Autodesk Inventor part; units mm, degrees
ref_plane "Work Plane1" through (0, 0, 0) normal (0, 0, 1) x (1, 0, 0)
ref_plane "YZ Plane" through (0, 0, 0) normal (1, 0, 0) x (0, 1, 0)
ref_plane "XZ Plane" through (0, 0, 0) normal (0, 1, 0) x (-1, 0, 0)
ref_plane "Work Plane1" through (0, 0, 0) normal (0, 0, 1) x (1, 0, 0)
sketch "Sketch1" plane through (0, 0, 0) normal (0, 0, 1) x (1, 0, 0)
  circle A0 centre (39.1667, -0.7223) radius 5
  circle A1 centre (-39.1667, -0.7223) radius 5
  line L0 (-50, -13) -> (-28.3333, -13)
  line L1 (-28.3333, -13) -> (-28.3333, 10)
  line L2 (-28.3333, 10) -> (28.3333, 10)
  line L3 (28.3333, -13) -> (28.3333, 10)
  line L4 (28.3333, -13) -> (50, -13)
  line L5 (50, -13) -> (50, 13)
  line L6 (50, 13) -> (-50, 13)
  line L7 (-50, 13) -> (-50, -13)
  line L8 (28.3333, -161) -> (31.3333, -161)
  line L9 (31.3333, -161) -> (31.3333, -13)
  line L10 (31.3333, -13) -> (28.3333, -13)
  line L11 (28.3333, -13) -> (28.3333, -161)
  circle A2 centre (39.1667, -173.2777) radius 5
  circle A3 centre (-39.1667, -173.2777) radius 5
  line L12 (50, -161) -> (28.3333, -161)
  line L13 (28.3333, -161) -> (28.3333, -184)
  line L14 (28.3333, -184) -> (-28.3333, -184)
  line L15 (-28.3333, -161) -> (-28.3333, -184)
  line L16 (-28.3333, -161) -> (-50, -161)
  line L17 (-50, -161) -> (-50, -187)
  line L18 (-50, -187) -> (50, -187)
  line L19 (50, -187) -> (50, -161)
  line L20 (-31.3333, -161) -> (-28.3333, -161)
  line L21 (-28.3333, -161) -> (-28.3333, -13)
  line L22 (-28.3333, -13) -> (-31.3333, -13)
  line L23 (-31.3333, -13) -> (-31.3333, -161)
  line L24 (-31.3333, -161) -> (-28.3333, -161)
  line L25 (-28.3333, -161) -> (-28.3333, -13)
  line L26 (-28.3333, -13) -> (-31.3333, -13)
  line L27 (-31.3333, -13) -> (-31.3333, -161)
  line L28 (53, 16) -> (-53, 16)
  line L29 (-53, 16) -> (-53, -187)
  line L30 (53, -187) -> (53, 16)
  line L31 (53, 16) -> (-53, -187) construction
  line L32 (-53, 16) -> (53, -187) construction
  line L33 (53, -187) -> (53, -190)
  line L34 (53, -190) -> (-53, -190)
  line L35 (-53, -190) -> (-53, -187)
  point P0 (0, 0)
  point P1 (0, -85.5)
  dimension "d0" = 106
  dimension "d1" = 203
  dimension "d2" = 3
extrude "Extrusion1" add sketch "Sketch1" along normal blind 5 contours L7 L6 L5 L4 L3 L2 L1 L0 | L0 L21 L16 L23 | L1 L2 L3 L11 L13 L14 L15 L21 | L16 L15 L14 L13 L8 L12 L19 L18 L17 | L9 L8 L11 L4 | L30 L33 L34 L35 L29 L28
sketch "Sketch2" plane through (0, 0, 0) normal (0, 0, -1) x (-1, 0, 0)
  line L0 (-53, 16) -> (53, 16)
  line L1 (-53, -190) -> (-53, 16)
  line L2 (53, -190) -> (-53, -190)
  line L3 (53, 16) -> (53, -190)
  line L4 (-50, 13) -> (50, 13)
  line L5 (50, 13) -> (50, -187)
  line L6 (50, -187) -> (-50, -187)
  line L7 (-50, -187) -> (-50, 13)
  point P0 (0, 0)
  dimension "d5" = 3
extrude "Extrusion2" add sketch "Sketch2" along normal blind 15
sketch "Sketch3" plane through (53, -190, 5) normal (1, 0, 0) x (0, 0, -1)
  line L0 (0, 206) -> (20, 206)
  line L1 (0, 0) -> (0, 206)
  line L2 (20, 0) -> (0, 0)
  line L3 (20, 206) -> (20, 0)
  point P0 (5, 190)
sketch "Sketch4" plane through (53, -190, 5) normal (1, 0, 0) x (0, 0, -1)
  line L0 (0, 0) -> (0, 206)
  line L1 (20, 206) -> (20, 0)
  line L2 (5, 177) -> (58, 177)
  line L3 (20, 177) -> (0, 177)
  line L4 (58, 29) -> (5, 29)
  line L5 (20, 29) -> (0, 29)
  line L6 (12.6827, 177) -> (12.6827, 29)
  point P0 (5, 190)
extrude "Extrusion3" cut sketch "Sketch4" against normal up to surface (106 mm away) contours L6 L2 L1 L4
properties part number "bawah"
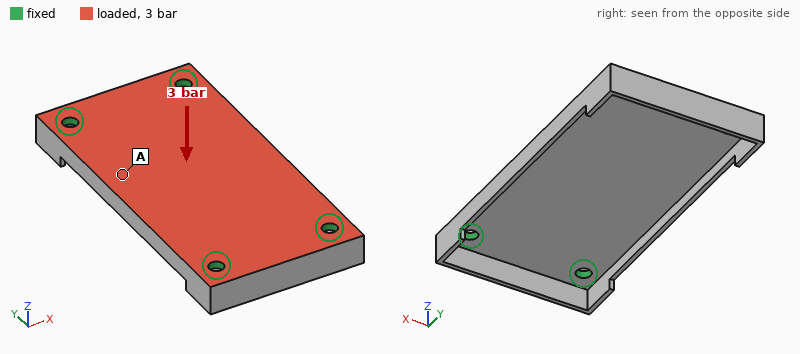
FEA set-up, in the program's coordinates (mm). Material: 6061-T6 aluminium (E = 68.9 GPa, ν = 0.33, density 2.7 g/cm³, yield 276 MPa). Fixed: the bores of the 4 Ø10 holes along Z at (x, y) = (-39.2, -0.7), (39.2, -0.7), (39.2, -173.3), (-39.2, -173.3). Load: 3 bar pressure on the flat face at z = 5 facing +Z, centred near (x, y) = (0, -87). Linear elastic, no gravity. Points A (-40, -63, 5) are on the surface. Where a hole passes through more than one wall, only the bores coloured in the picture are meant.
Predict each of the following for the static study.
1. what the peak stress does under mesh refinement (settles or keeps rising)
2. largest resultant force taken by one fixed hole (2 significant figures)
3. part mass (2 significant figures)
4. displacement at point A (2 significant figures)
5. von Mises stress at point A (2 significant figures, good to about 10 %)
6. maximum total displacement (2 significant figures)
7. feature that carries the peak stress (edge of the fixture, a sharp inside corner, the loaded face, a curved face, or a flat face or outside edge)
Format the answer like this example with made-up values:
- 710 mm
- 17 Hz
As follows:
- keeps rising
- 1.6 kN
- 350 g
- 0.40 mm
- 36 MPa
- 0.56 mm
- edge of the fixture
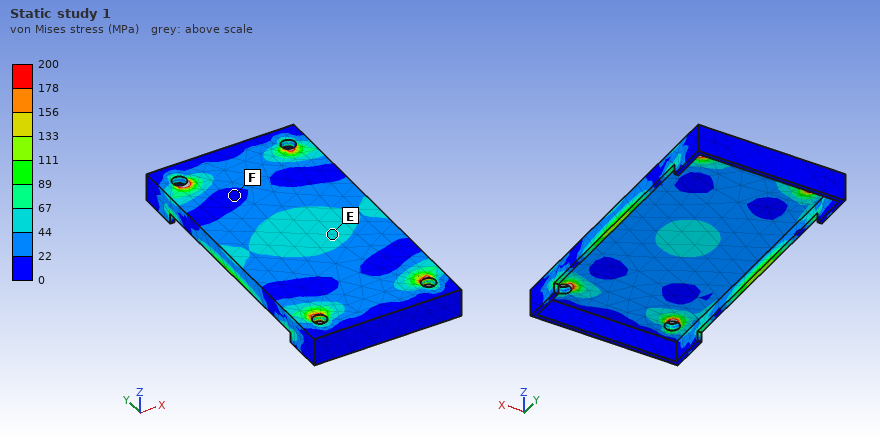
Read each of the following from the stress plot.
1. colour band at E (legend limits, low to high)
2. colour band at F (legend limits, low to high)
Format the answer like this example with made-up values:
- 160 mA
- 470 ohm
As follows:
- 44 to 67 MPa
- 0 to 22 MPa
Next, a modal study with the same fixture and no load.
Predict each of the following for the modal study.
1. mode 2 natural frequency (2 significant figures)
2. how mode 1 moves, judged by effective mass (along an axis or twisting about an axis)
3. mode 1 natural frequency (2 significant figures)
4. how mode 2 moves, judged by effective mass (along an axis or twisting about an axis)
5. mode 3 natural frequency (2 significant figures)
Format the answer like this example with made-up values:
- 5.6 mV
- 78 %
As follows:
- 1700 Hz
- along Z
- 1200 Hz
- twisting about Y
- 2800 Hz
